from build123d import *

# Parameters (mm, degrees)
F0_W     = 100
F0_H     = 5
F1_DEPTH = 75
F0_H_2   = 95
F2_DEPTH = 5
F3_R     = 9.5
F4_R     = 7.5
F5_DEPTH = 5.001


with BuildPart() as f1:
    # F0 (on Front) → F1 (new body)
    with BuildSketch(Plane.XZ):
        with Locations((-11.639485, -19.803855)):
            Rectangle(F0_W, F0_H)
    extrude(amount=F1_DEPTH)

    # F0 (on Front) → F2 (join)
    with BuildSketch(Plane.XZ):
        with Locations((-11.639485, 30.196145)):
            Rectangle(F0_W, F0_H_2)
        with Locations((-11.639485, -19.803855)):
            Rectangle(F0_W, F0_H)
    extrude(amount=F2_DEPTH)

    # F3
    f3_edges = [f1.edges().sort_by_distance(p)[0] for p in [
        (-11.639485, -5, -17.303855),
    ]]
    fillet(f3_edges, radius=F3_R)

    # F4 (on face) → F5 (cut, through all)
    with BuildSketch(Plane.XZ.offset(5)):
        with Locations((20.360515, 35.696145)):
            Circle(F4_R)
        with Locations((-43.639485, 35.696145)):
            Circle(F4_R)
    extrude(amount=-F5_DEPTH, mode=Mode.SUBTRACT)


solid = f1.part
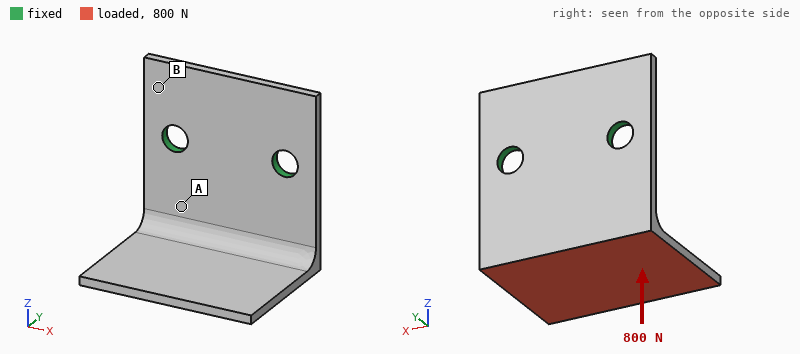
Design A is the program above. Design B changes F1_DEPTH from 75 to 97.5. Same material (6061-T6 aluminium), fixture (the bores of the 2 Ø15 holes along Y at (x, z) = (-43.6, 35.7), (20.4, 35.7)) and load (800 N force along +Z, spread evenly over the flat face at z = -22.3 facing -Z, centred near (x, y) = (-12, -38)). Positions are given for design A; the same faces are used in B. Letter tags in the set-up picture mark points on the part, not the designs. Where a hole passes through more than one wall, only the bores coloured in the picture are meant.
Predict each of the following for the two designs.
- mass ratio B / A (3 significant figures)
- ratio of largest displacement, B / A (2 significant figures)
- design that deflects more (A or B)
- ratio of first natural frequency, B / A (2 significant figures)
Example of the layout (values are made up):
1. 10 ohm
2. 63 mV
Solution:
1. 1.13
2. 1.8
3. B
4. 0.70
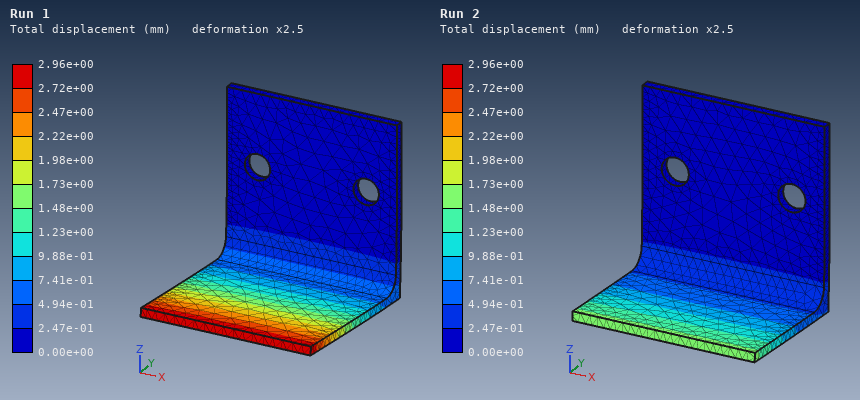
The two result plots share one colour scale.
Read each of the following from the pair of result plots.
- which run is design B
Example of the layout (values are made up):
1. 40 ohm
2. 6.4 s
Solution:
1. Run 1
